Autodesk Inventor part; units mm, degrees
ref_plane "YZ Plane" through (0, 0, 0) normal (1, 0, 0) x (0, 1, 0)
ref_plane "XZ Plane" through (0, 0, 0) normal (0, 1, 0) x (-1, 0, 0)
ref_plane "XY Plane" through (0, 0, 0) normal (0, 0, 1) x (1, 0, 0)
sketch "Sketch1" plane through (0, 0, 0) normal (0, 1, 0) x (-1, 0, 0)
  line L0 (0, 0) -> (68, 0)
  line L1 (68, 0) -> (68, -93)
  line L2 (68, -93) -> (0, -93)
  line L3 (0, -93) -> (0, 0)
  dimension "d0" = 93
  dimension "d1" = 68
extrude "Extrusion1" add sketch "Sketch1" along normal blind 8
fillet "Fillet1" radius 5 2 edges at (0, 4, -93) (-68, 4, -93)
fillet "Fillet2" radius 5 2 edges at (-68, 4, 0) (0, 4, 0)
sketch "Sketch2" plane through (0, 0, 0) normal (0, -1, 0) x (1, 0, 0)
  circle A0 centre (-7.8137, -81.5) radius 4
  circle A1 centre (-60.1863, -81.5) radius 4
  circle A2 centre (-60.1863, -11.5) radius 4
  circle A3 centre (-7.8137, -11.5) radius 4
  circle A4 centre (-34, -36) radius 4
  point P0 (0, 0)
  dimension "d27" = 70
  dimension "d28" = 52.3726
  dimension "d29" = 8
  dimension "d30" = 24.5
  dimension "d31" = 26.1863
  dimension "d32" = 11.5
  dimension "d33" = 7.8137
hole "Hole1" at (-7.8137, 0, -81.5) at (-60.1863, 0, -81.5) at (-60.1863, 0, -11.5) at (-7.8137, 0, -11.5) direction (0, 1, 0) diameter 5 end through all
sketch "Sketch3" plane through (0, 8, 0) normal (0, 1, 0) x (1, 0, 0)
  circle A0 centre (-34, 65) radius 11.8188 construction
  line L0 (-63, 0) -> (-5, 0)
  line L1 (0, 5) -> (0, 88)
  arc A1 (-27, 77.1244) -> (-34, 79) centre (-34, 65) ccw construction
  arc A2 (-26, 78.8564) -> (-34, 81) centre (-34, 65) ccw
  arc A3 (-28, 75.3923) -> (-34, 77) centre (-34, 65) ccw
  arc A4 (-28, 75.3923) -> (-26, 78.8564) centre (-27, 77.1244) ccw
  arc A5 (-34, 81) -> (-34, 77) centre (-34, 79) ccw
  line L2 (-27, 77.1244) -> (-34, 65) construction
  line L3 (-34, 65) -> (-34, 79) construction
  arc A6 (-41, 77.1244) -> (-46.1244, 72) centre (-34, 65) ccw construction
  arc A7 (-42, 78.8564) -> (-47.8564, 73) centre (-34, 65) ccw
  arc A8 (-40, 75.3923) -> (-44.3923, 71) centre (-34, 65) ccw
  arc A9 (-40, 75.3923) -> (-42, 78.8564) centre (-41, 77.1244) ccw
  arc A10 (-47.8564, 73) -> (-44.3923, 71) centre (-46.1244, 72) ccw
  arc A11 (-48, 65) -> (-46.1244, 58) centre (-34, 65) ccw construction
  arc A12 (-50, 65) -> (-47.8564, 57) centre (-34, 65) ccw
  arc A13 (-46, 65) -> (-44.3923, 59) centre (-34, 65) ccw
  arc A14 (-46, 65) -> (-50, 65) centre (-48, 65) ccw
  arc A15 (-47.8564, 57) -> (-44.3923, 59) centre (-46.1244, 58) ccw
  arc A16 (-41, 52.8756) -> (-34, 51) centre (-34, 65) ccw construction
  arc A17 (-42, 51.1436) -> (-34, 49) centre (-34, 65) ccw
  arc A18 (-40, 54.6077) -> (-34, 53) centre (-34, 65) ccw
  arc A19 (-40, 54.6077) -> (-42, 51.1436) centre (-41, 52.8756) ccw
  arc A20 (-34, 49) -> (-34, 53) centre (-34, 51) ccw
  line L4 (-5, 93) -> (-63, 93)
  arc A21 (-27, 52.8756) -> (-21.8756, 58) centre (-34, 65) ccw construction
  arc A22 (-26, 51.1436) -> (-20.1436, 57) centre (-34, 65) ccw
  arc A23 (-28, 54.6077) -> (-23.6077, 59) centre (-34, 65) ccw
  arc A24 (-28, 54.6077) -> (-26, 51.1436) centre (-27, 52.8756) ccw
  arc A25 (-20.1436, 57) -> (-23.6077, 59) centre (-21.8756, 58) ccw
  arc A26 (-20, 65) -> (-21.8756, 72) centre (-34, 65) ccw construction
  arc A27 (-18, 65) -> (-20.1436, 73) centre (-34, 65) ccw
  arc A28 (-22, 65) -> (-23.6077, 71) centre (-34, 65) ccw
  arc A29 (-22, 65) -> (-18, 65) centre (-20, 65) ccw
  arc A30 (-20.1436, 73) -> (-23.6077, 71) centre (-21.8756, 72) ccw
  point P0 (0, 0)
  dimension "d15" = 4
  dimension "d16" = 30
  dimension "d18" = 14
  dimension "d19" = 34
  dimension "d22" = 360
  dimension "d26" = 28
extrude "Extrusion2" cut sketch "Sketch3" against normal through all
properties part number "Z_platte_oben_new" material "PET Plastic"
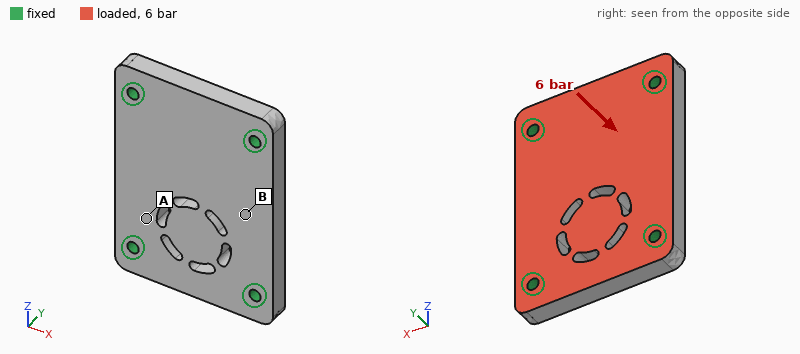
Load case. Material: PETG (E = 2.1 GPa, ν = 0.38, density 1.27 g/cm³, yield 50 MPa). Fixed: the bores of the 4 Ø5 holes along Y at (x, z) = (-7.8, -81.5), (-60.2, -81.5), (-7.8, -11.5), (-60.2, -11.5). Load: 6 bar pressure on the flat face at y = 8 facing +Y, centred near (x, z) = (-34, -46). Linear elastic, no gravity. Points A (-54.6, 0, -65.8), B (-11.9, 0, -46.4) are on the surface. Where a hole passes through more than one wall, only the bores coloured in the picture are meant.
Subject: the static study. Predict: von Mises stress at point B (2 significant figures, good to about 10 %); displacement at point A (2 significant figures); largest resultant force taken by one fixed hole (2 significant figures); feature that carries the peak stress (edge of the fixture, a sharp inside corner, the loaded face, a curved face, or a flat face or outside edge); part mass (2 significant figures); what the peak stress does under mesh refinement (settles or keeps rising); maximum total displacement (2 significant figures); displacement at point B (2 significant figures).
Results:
13 MPa
0.40 mm
920 N
edge of the fixture
61 g
keeps rising
0.83 mm
0.64 mm
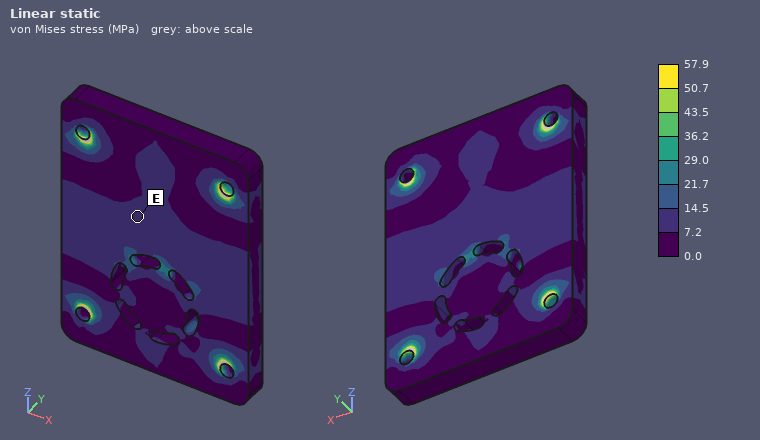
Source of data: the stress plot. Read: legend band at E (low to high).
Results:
7.2 to 14.5 MPa
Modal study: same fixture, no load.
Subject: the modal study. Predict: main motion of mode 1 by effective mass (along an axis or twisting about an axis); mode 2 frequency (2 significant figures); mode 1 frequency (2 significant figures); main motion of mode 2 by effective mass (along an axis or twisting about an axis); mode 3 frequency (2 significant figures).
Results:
along Y
2300 Hz
1600 Hz
twisting about Z
3000 Hz
